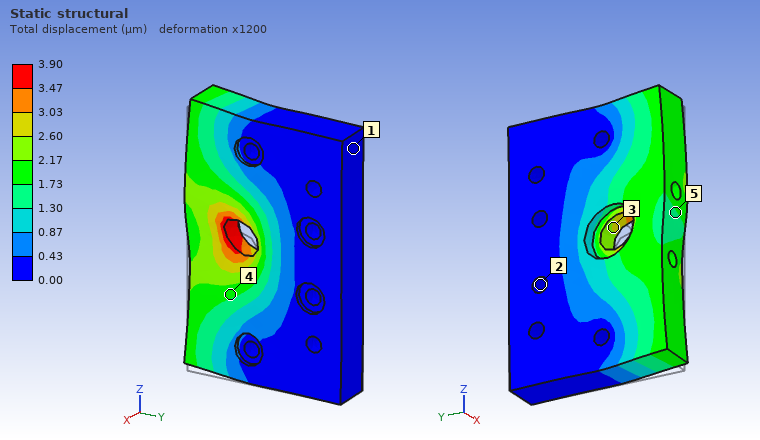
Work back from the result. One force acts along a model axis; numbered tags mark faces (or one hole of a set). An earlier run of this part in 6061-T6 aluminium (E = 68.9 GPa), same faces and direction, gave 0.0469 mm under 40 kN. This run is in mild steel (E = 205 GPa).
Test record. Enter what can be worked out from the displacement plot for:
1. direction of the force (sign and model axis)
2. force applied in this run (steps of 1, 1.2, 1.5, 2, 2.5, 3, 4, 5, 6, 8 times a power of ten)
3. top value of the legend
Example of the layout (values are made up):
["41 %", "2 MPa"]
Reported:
["+Z", "10 kN", "3.90 µm"]
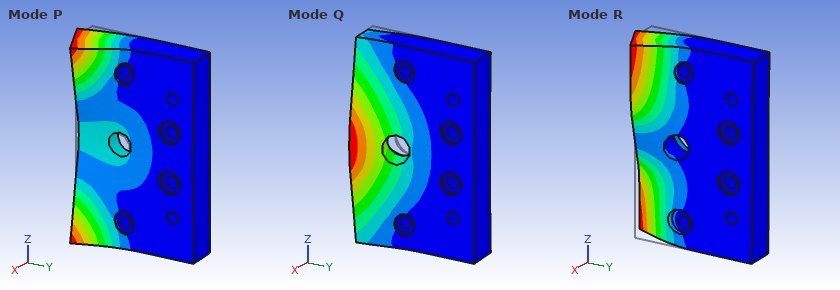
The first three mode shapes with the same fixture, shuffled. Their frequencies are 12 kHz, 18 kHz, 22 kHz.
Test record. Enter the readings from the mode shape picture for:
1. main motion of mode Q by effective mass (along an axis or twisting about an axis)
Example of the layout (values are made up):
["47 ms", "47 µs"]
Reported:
["along X"]
